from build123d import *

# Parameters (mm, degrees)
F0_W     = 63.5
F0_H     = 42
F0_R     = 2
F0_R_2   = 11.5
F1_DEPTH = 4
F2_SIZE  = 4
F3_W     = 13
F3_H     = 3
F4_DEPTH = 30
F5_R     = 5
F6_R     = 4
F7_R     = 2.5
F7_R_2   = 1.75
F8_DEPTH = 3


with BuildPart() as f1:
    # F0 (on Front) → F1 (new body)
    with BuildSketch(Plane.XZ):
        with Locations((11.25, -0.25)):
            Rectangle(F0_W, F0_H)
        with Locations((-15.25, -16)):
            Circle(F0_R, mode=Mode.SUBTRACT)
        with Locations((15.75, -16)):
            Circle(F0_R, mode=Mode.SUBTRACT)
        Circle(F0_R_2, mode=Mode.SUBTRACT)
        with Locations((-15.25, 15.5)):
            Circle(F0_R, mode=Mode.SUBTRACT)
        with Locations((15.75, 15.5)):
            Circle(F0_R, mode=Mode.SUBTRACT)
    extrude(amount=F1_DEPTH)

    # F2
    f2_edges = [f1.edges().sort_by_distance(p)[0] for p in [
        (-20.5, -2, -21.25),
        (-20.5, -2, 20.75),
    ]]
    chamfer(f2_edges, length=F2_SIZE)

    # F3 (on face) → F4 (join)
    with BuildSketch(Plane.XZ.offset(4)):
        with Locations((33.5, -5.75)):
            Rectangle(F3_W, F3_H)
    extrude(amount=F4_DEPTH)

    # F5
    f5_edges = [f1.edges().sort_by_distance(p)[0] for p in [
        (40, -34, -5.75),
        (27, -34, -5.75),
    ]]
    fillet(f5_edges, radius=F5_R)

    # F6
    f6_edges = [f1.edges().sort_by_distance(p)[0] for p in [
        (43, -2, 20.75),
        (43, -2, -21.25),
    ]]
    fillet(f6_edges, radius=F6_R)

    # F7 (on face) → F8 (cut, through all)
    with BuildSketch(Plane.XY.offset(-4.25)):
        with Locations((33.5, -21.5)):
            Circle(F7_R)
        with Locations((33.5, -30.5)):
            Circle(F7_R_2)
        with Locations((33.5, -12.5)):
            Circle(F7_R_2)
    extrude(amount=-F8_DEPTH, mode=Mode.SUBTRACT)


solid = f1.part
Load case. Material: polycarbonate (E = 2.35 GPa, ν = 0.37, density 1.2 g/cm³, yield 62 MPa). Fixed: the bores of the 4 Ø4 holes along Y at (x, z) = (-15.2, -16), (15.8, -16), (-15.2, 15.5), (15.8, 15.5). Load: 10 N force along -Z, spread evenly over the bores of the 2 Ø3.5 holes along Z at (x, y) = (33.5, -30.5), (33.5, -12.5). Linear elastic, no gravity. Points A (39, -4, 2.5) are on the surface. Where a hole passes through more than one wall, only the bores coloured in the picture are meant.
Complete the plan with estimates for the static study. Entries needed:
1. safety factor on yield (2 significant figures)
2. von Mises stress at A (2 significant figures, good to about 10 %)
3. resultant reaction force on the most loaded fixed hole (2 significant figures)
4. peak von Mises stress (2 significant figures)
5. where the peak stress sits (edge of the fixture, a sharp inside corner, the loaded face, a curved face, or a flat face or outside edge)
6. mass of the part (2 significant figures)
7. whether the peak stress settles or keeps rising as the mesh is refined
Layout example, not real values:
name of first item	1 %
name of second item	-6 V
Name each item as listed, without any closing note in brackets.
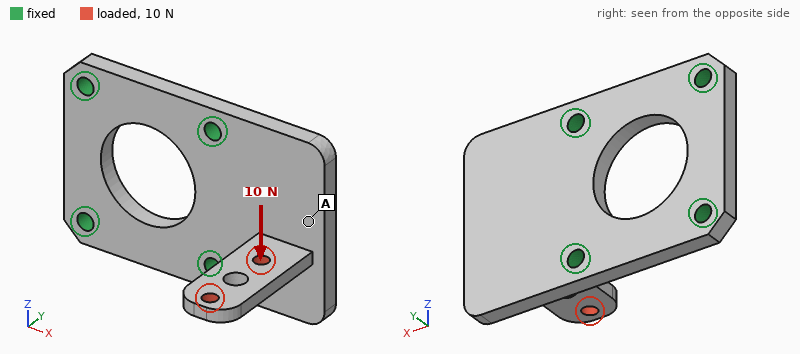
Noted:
safety factor on yield	6.3
von Mises stress at A	1.3 MPa
resultant reaction force on the most loaded fixed hole	9.7 N
peak von Mises stress	9.9 MPa
where the peak stress sits	the loaded face
mass of the part	12 g
whether the peak stress settles or keeps rising as the mesh is refined	settles
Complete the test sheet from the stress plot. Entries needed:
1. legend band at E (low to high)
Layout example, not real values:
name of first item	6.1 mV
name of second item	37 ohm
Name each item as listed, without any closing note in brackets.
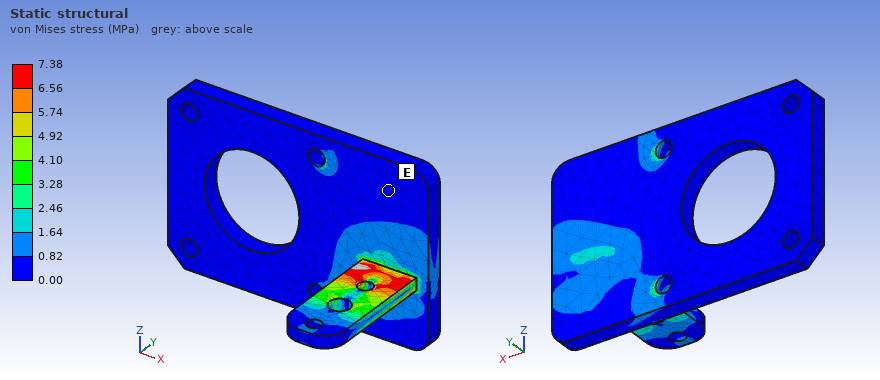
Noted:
legend band at E	0.00 to 0.82 MPa
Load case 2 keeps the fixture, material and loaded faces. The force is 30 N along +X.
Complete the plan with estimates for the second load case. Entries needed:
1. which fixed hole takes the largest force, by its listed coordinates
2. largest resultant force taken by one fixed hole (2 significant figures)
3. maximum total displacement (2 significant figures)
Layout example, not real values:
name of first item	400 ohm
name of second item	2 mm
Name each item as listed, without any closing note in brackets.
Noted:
which fixed hole takes the largest force, by its listed coordinates	(15.8, -16)
largest resultant force taken by one fixed hole	20 N
maximum total displacement	0.85 mm
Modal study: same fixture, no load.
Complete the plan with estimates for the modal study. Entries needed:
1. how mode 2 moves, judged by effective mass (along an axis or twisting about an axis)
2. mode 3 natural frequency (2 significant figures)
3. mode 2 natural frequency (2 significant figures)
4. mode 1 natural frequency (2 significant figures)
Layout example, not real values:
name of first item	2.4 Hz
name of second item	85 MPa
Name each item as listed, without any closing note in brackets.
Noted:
how mode 2 moves, judged by effective mass	along Y
mode 3 natural frequency	2100 Hz
mode 2 natural frequency	800 Hz
mode 1 natural frequency	710 Hz
